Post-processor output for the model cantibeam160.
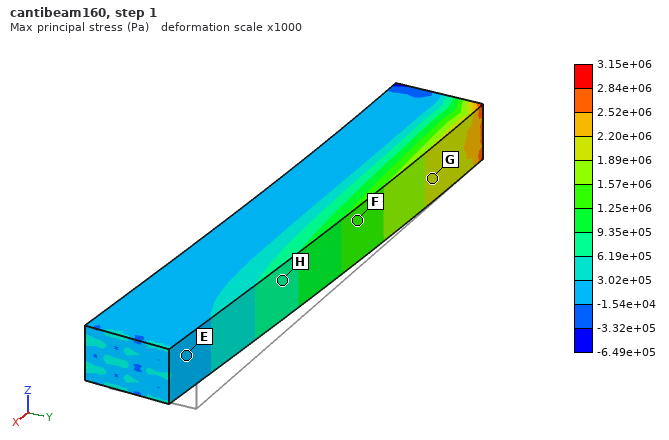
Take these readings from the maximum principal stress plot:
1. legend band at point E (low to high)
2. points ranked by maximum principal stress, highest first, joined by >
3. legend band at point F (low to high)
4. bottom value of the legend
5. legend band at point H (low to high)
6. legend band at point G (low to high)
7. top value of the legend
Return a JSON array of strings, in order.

["-1.54e+04 to 3.02e+05 Pa", "G > F > H > E", "1.25e+06 to 1.57e+06 Pa", "-6.49e+05 Pa", "6.19e+05 to 9.35e+05 Pa", "1.89e+06 to 2.20e+06 Pa", "3.15e+06 Pa"]
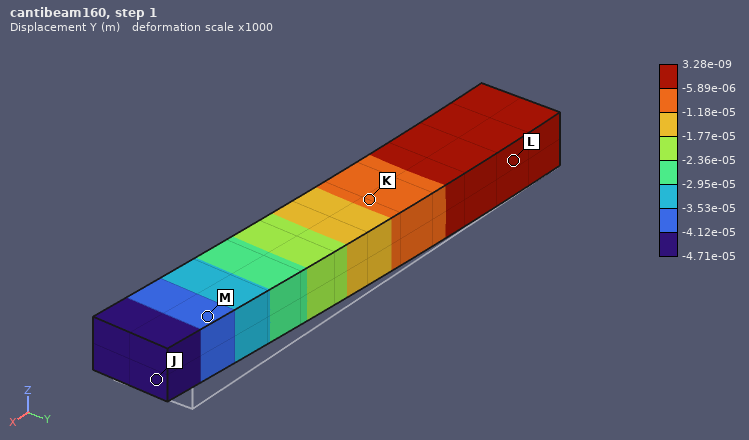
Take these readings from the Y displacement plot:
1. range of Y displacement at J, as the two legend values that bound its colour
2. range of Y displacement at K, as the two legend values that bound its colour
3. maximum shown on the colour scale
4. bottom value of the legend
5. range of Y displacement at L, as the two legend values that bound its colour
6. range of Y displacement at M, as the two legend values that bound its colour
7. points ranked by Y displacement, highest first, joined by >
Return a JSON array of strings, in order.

["-4.71e-05 to -4.12e-05 m", "-1.18e-05 to -5.89e-06 m", "3.28e-09 m", "-4.71e-05 m", "-5.89e-06 to 3.28e-09 m", "-4.12e-05 to -3.53e-05 m", "L > K > M > J"]
